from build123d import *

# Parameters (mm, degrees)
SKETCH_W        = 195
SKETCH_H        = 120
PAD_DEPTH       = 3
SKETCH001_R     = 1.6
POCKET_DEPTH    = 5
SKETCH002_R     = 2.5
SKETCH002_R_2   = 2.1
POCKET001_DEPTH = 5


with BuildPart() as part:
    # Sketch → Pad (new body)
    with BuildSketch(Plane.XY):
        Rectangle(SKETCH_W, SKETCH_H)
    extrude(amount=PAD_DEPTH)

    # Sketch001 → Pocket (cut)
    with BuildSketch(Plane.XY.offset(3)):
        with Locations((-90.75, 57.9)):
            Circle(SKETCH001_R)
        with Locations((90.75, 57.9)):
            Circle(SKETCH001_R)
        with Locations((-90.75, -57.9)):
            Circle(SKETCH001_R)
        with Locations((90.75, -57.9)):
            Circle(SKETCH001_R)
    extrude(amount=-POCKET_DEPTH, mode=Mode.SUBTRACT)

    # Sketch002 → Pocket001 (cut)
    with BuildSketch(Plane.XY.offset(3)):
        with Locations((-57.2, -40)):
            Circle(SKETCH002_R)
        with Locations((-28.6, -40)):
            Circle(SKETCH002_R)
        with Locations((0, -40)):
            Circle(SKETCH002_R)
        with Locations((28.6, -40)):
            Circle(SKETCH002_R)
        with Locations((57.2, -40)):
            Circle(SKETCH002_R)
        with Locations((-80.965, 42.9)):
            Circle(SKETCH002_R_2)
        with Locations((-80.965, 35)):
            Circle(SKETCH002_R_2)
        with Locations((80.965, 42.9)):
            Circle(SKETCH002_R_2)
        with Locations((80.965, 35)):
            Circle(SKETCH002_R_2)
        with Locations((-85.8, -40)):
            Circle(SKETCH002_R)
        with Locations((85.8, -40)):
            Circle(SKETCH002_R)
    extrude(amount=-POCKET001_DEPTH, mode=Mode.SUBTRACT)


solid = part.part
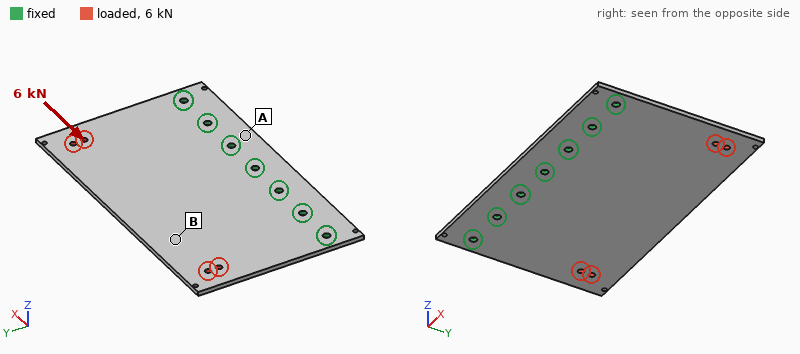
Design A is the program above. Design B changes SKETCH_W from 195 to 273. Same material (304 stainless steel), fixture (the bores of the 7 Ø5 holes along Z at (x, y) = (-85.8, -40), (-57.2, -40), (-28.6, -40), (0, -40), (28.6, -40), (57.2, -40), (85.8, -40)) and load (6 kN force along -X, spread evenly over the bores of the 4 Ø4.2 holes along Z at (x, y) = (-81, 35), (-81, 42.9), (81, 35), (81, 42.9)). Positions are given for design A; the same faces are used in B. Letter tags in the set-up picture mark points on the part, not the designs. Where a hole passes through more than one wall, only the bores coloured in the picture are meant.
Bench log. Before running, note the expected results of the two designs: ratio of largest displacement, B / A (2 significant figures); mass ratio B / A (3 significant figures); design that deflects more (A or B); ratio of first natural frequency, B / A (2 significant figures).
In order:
1.1
1.40
B
0.93
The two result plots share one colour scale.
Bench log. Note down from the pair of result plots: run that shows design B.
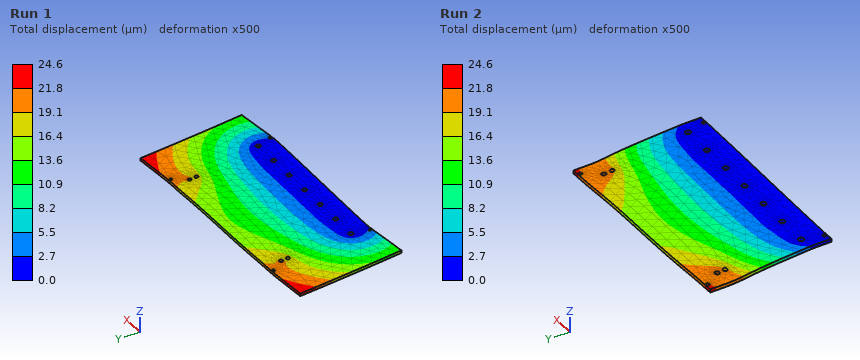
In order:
Run 1
